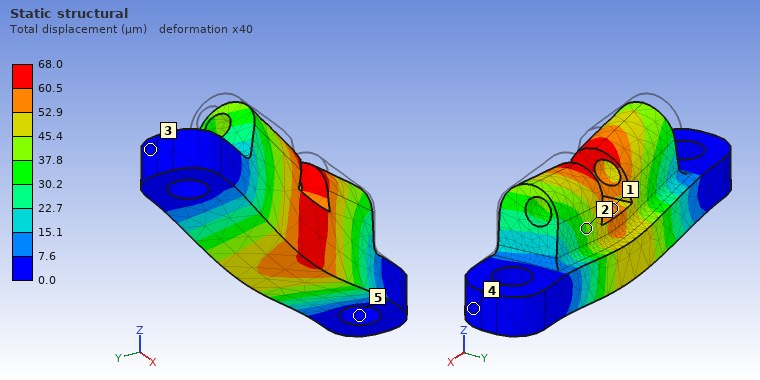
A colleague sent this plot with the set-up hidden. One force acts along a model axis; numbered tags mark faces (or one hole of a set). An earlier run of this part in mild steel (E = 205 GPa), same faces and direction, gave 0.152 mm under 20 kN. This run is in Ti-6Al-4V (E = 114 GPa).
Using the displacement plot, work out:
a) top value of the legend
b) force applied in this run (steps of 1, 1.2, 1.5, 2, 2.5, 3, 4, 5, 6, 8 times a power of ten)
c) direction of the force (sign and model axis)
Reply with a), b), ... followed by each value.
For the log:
a) 68.0 µm
b) 5 kN
c) -Z
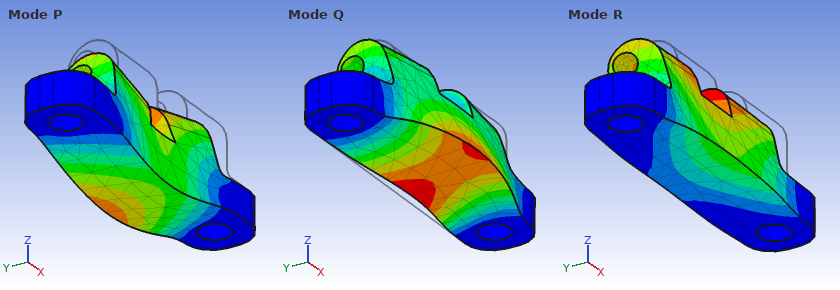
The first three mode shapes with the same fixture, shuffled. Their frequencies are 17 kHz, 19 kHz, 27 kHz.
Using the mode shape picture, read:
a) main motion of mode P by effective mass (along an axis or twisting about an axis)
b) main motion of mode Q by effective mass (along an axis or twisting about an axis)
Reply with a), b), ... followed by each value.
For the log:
a) along Z
b) along Y
